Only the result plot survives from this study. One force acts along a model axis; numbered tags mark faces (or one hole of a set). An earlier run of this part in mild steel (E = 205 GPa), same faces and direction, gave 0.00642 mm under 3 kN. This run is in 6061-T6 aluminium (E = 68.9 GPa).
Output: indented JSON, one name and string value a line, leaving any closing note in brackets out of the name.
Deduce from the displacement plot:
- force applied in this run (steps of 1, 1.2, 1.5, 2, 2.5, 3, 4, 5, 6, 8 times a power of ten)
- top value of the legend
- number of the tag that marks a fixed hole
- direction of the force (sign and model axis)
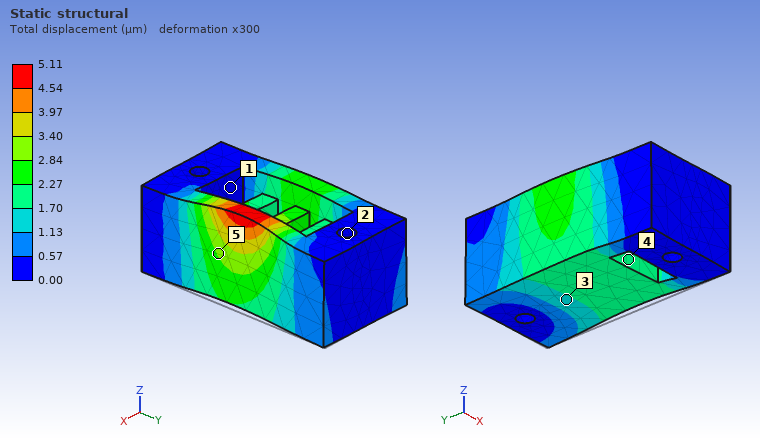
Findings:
{
  "force applied in this run": "800 N",
  "top value of the legend": "5.11 µm",
  "number of the tag that marks a fixed hole": "2",
  "direction of the force": "-X"
}
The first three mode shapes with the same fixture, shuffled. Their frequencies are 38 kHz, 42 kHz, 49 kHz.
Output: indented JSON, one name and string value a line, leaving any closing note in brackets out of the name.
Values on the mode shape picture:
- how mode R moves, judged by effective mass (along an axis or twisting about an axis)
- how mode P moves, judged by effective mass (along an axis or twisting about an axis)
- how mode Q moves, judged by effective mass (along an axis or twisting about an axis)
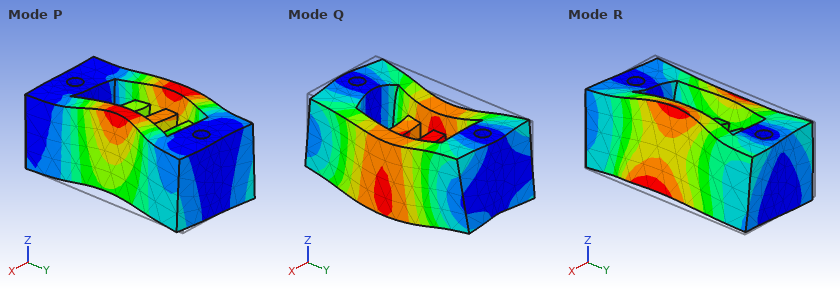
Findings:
{
  "how mode R moves, judged by effective mass": "twisting about Y",
  "how mode P moves, judged by effective mass": "along X",
  "how mode Q moves, judged by effective mass": "along Z"
}
